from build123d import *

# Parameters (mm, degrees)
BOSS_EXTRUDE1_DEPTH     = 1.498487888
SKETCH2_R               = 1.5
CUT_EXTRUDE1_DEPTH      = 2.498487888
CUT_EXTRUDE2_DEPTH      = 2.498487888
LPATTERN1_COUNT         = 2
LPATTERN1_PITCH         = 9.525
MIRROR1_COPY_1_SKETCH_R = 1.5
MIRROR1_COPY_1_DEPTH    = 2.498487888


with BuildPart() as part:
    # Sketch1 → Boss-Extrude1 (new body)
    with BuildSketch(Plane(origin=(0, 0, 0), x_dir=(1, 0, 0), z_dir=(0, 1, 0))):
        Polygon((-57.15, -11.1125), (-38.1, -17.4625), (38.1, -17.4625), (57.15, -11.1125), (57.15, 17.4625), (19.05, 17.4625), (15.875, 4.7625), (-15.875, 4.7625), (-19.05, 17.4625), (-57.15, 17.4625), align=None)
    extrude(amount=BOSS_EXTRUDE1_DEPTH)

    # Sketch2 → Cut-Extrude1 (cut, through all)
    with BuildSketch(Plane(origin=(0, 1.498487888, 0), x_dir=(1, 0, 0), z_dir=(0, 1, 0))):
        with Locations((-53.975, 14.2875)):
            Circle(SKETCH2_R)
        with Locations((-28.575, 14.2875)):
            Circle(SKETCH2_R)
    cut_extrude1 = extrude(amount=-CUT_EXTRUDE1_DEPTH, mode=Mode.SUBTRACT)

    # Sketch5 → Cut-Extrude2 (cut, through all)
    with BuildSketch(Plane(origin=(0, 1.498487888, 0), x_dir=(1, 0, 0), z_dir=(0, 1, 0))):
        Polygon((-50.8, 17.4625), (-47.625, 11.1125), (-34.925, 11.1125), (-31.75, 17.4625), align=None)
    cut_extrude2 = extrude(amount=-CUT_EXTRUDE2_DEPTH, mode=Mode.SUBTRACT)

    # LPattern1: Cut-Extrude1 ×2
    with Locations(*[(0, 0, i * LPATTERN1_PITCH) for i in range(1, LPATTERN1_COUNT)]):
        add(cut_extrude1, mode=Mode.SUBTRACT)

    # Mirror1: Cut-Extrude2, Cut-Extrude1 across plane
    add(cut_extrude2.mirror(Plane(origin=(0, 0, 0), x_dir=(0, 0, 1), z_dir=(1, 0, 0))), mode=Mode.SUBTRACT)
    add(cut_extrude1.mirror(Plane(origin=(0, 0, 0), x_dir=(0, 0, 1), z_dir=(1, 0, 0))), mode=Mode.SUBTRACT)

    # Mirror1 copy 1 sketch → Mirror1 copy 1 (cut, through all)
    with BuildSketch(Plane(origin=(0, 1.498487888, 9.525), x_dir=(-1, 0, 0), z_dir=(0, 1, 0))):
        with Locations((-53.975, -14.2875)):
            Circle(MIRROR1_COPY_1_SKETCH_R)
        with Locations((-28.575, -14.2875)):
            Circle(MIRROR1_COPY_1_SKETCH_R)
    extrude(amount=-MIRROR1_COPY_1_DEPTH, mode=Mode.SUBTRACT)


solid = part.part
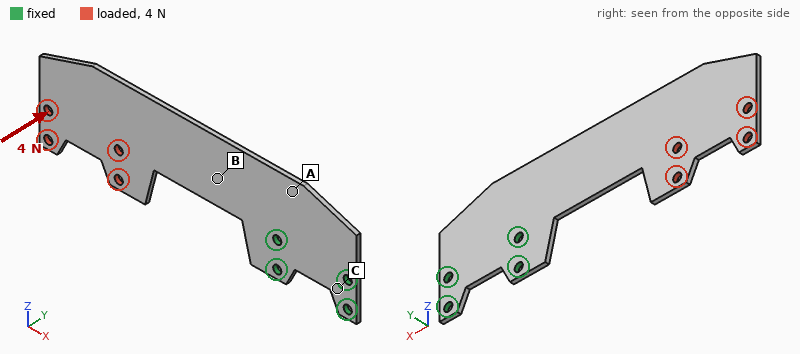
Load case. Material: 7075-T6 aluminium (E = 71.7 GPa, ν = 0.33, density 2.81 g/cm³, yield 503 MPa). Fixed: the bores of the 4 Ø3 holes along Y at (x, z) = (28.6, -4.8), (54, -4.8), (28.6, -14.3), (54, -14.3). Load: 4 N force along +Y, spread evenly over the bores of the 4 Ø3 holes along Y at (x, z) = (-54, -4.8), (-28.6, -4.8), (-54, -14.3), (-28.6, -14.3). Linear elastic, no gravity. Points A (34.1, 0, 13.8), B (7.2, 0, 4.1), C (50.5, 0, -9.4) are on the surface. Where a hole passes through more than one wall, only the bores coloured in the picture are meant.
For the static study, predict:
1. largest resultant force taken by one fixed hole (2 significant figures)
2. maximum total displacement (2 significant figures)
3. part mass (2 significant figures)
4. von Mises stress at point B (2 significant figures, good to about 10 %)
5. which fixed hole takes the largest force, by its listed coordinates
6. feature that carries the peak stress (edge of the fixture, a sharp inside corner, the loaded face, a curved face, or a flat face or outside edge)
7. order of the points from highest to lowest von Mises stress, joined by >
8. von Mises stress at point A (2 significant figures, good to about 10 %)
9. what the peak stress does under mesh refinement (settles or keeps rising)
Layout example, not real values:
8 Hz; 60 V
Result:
8.6 N; 1.4 mm; 13 g; 25 MPa; (28.6, -4.8); edge of the fixture; B > A > C; 8.5 MPa; keeps rising
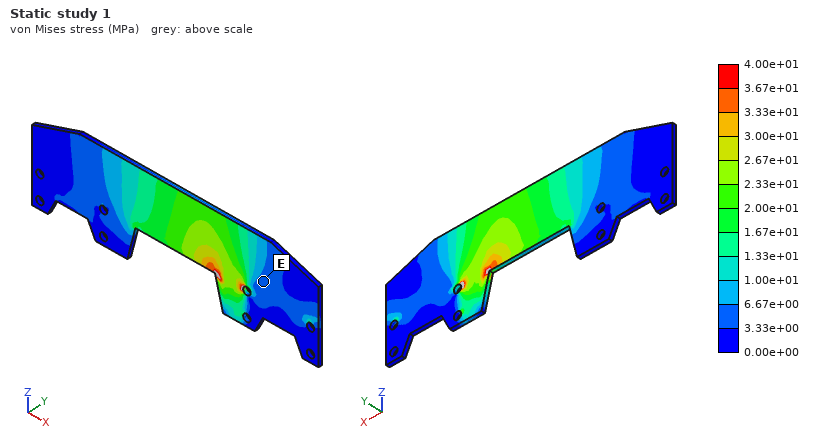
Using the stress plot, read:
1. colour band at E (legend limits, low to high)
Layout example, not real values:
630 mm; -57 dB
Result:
3.33e+00 to 6.67e+00 MPa
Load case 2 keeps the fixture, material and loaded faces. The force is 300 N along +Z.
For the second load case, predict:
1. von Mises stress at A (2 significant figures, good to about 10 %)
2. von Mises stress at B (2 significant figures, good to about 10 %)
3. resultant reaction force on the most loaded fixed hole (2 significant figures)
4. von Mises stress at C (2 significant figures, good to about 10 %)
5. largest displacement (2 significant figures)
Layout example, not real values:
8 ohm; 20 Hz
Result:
52 MPa; 32 MPa; 660 N; 14 MPa; 0.53 mm
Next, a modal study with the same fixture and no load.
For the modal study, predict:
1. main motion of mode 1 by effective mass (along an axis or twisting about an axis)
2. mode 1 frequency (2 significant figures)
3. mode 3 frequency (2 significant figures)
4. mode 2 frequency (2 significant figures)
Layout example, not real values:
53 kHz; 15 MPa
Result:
along Y; 150 Hz; 1000 Hz; 740 Hz
